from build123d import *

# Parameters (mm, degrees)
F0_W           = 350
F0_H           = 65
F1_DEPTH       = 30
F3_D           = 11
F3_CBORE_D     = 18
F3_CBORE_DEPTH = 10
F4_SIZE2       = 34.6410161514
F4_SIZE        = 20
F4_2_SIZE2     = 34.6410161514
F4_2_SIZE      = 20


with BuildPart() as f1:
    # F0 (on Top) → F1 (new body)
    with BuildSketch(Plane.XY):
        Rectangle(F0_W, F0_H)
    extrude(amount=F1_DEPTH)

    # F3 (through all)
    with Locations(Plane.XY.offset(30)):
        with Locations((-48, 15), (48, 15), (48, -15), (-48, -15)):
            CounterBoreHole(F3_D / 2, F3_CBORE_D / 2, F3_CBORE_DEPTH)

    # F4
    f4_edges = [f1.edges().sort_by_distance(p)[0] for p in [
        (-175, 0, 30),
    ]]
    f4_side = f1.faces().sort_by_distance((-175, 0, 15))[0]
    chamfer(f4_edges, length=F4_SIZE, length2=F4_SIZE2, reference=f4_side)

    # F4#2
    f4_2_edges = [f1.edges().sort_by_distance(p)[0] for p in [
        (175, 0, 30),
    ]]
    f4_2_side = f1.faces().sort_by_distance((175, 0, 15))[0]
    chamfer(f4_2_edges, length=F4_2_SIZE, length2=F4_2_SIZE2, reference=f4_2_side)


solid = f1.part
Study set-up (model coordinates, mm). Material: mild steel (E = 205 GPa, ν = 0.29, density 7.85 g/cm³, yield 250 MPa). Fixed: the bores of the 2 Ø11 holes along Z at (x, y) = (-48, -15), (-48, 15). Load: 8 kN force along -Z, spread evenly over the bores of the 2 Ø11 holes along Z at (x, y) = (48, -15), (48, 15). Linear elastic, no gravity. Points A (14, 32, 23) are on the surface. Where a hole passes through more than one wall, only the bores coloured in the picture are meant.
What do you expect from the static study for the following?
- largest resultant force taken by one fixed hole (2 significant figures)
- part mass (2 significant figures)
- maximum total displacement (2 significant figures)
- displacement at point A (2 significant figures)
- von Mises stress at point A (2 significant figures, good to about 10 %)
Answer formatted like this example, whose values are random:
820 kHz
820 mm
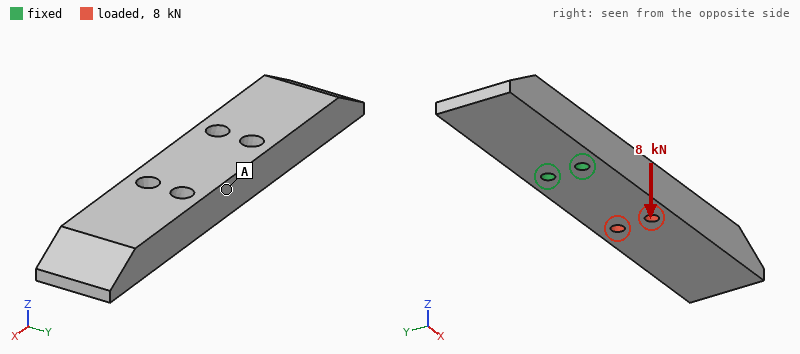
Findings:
4.1 kN
4.9 kg
0.32 mm
0.064 mm
18 MPa
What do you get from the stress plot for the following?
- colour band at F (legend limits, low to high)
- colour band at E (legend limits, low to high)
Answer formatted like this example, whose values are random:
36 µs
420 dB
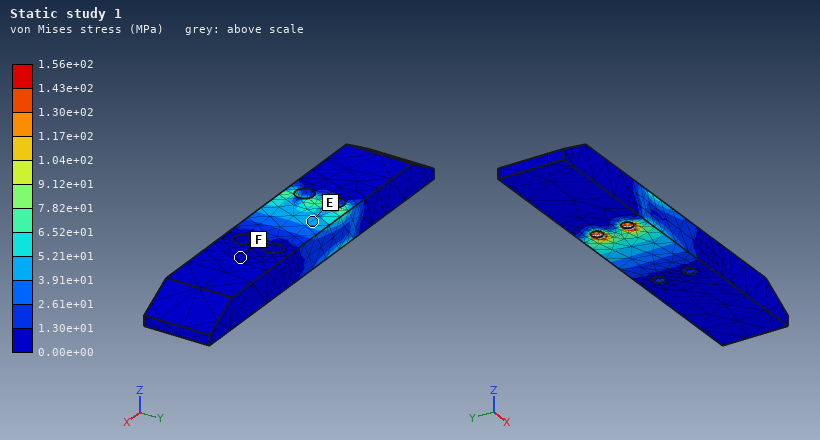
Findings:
0.00e+00 to 1.30e+01 MPa
3.91e+01 to 5.21e+01 MPa
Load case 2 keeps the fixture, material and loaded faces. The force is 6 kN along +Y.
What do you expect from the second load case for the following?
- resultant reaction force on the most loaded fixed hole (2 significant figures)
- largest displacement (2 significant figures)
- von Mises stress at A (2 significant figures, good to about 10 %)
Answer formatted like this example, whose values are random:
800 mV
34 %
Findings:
16 kN
57 µm
9.5 MPa
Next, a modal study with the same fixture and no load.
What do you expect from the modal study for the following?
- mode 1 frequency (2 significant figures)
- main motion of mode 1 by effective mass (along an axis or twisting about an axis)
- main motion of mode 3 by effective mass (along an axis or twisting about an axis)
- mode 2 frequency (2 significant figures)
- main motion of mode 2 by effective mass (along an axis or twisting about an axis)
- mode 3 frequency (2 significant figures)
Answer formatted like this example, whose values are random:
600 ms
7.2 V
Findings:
470 Hz
along Z
along Z
990 Hz
along Y
1500 Hz
